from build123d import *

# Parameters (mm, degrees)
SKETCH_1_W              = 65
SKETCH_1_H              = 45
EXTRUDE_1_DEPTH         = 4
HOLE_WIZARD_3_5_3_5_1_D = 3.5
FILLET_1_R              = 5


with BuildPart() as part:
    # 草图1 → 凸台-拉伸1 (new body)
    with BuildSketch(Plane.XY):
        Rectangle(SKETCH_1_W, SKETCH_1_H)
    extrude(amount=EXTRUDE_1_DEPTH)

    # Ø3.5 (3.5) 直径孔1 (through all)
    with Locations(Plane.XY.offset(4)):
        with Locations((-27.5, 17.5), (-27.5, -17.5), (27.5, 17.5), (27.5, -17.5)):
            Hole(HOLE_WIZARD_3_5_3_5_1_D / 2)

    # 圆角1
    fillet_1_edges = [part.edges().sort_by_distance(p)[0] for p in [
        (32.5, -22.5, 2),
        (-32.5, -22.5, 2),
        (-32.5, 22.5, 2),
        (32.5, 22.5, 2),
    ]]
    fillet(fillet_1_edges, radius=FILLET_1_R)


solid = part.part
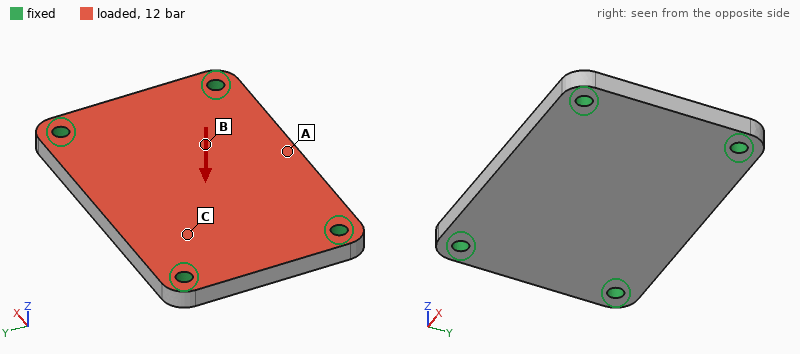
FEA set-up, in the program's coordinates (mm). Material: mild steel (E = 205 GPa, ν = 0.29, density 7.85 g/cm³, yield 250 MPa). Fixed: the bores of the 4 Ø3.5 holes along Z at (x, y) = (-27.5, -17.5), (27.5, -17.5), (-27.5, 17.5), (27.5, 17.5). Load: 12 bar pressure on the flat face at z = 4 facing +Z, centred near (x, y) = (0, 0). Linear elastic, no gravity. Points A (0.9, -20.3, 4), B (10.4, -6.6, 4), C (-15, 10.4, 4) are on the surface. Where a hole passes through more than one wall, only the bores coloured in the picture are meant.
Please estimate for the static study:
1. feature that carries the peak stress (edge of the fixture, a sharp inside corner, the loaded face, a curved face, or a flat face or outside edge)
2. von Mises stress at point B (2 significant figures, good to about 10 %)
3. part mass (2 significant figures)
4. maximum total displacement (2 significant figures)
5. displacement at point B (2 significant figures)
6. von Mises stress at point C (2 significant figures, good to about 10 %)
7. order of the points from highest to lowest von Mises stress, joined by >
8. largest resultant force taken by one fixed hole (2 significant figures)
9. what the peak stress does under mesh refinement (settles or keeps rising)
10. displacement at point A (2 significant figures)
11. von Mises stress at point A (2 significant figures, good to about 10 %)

edge of the fixture
38 MPa
90 g
38 µm
30 µm
21 MPa
A > B > C
860 N
keeps rising
34 µm
69 MPa
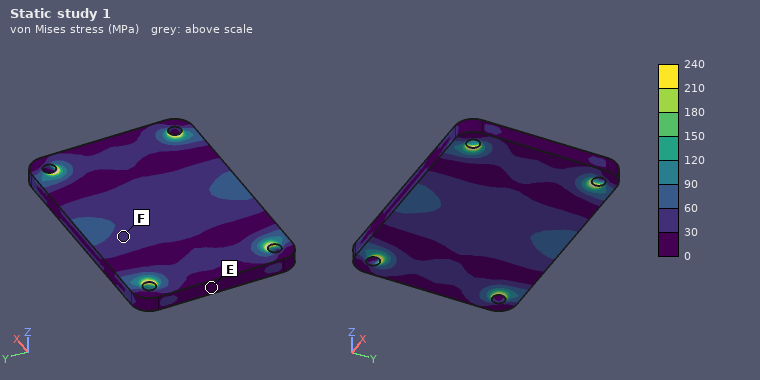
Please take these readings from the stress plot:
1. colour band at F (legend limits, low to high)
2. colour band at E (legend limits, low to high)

30 to 60 MPa
0 to 30 MPa
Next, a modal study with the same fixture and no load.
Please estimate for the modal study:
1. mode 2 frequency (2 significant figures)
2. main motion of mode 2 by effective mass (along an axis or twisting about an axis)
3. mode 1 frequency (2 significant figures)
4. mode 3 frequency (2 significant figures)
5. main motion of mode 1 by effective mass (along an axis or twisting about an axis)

8700 Hz
twisting about X
5900 Hz
14 kHz
along Z
